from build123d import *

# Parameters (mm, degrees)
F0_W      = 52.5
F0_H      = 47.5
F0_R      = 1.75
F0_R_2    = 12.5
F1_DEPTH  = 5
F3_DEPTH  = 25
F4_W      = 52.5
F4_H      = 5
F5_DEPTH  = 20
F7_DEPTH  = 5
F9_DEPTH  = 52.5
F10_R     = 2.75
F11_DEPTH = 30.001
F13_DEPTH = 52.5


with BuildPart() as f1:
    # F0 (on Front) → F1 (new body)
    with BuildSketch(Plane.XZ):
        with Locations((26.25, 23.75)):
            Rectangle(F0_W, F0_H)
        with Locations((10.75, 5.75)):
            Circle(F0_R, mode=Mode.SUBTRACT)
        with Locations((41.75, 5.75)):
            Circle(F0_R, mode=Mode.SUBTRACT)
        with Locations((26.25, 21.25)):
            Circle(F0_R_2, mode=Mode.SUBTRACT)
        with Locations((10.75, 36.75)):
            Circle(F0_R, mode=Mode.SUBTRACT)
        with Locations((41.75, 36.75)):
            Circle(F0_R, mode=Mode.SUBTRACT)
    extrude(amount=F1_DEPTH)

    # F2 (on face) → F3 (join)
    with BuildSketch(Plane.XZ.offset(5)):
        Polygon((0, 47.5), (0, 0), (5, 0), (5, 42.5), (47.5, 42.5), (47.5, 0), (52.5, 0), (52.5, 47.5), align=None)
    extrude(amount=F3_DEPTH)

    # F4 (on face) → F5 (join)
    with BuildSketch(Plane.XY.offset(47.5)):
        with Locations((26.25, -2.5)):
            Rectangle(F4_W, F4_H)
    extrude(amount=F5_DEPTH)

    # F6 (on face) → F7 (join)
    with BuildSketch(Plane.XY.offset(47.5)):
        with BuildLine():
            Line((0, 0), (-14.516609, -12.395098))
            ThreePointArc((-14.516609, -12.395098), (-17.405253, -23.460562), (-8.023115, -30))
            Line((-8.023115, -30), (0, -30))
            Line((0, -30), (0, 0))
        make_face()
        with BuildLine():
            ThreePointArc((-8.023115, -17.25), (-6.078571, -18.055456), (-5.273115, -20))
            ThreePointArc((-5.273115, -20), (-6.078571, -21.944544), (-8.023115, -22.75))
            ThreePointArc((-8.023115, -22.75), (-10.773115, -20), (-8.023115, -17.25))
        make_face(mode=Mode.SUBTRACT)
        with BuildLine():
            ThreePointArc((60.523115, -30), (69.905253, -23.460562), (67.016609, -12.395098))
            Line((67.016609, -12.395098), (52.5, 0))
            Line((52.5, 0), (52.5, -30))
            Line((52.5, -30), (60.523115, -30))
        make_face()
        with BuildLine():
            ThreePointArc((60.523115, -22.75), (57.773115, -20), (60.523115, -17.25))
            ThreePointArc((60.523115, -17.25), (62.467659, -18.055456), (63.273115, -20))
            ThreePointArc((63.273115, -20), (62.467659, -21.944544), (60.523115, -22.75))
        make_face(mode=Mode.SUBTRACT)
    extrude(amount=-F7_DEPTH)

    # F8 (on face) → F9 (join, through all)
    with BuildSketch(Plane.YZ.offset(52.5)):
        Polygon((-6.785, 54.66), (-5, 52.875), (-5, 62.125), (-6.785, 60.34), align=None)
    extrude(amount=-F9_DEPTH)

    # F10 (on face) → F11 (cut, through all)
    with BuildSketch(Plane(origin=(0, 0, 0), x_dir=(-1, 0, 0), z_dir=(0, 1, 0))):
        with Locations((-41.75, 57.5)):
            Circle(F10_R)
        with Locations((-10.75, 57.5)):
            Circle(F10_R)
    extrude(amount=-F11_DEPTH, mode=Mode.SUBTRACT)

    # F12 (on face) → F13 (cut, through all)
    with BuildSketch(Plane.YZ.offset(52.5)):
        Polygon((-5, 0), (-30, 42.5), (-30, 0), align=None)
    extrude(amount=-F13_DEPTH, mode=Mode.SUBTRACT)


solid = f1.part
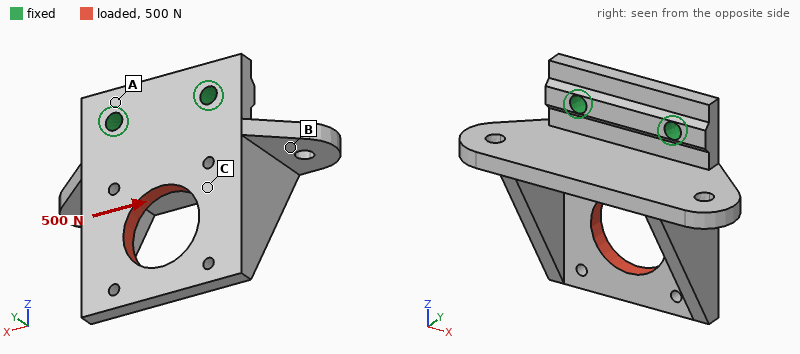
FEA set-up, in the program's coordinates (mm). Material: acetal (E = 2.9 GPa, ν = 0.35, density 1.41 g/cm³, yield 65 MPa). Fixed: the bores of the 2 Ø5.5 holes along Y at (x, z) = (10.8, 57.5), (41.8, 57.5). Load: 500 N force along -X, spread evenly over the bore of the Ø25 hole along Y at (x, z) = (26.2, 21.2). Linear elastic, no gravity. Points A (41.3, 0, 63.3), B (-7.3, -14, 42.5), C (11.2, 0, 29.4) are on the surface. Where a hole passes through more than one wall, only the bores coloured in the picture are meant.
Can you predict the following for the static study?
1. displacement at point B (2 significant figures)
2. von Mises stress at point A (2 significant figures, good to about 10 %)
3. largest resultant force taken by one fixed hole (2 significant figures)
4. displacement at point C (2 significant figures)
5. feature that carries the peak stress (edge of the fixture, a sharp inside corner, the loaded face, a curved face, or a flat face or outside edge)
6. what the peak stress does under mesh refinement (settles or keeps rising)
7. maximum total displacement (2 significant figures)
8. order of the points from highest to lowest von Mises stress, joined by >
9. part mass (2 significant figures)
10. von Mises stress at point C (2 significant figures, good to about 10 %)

0.11 mm
2.3 MPa
570 N
0.12 mm
edge of the fixture
keeps rising
0.31 mm
C > A > B
44 g
4.5 MPa
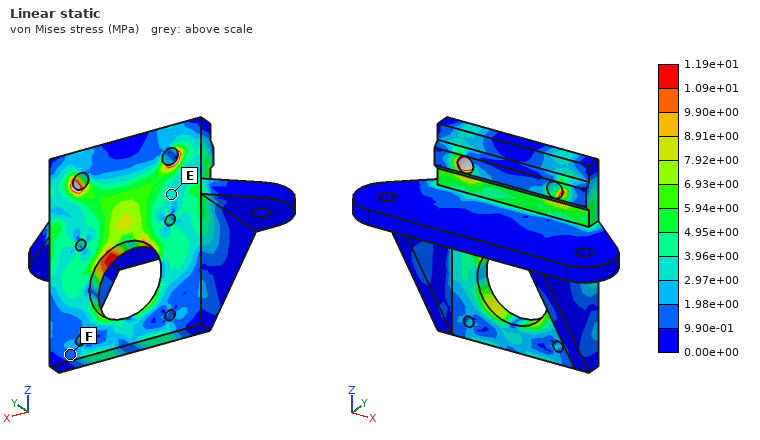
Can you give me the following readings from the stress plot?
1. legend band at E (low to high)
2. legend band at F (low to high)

2.97e+00 to 3.96e+00 MPa
9.90e-01 to 1.98e+00 MPa
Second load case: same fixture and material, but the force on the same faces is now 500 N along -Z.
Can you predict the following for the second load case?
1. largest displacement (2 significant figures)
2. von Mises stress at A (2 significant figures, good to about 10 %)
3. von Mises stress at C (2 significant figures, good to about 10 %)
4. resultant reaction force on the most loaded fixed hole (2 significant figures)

98 µm
0.85 MPa
3.0 MPa
250 N
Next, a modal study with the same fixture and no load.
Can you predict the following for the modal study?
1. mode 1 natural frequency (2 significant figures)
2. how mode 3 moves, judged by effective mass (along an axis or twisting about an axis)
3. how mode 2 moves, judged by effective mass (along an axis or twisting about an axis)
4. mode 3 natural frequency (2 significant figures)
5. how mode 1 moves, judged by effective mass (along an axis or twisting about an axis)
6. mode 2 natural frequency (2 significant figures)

390 Hz
along X
twisting about Z
1600 Hz
along Y
810 Hz
